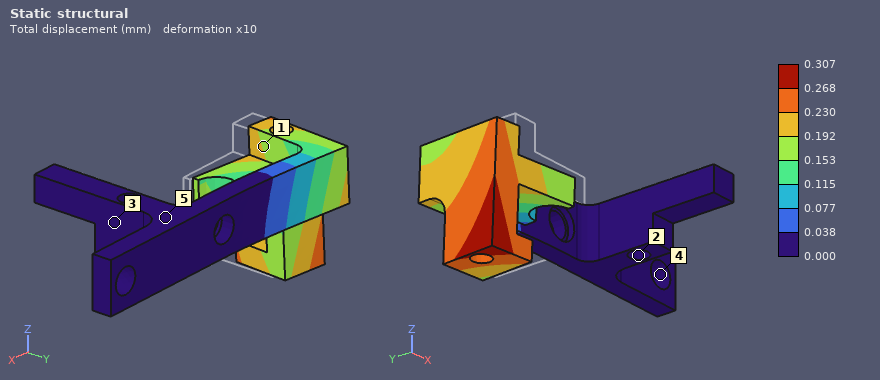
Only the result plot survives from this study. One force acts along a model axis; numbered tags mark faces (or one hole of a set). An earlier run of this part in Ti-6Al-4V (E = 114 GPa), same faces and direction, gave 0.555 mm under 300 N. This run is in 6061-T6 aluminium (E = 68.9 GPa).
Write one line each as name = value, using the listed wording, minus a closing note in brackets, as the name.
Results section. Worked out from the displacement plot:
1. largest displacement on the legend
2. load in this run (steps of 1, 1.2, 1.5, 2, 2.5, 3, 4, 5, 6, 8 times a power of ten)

largest displacement on the legend = 0.307 mm
load in this run = 100 N
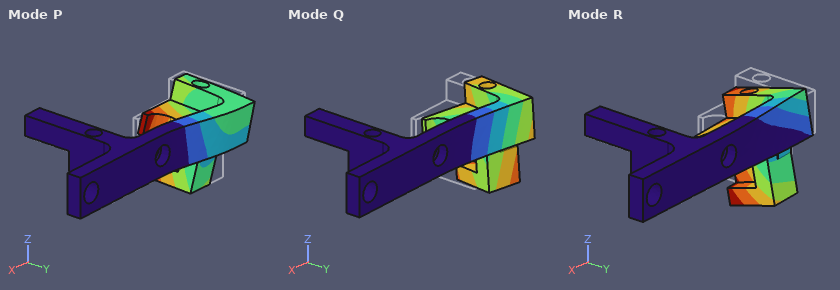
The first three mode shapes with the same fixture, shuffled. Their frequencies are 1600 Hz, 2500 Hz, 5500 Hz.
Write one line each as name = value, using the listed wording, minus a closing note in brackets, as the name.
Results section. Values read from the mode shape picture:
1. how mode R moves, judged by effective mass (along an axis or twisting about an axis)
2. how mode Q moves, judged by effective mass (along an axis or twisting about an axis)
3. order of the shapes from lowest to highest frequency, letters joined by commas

how mode R moves, judged by effective mass = along Z
how mode Q moves, judged by effective mass = along Y
order of the shapes from lowest to highest frequency, letters joined by commas = Q, R, P
